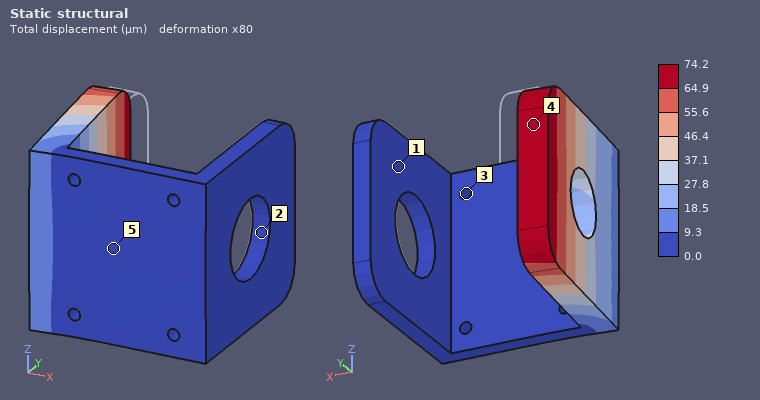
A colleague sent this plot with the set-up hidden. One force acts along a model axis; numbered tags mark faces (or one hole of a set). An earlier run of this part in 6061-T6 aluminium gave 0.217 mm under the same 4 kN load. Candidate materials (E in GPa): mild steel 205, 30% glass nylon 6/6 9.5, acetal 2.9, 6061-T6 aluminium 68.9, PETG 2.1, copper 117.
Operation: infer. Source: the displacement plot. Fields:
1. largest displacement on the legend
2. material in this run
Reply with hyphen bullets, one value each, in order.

- 74.2 µm
- mild steel
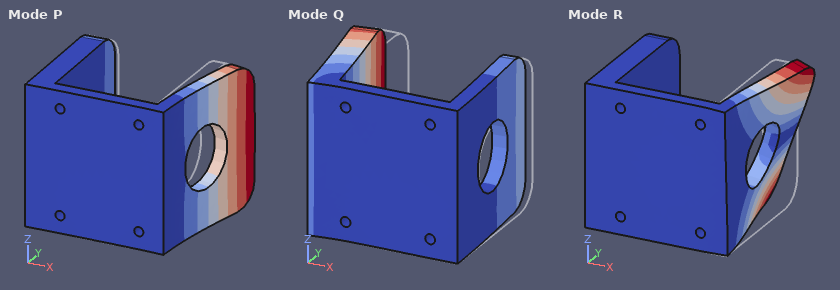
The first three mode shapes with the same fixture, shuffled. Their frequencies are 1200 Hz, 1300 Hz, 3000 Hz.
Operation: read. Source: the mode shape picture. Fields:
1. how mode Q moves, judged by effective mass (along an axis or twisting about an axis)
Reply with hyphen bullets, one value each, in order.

- along X
